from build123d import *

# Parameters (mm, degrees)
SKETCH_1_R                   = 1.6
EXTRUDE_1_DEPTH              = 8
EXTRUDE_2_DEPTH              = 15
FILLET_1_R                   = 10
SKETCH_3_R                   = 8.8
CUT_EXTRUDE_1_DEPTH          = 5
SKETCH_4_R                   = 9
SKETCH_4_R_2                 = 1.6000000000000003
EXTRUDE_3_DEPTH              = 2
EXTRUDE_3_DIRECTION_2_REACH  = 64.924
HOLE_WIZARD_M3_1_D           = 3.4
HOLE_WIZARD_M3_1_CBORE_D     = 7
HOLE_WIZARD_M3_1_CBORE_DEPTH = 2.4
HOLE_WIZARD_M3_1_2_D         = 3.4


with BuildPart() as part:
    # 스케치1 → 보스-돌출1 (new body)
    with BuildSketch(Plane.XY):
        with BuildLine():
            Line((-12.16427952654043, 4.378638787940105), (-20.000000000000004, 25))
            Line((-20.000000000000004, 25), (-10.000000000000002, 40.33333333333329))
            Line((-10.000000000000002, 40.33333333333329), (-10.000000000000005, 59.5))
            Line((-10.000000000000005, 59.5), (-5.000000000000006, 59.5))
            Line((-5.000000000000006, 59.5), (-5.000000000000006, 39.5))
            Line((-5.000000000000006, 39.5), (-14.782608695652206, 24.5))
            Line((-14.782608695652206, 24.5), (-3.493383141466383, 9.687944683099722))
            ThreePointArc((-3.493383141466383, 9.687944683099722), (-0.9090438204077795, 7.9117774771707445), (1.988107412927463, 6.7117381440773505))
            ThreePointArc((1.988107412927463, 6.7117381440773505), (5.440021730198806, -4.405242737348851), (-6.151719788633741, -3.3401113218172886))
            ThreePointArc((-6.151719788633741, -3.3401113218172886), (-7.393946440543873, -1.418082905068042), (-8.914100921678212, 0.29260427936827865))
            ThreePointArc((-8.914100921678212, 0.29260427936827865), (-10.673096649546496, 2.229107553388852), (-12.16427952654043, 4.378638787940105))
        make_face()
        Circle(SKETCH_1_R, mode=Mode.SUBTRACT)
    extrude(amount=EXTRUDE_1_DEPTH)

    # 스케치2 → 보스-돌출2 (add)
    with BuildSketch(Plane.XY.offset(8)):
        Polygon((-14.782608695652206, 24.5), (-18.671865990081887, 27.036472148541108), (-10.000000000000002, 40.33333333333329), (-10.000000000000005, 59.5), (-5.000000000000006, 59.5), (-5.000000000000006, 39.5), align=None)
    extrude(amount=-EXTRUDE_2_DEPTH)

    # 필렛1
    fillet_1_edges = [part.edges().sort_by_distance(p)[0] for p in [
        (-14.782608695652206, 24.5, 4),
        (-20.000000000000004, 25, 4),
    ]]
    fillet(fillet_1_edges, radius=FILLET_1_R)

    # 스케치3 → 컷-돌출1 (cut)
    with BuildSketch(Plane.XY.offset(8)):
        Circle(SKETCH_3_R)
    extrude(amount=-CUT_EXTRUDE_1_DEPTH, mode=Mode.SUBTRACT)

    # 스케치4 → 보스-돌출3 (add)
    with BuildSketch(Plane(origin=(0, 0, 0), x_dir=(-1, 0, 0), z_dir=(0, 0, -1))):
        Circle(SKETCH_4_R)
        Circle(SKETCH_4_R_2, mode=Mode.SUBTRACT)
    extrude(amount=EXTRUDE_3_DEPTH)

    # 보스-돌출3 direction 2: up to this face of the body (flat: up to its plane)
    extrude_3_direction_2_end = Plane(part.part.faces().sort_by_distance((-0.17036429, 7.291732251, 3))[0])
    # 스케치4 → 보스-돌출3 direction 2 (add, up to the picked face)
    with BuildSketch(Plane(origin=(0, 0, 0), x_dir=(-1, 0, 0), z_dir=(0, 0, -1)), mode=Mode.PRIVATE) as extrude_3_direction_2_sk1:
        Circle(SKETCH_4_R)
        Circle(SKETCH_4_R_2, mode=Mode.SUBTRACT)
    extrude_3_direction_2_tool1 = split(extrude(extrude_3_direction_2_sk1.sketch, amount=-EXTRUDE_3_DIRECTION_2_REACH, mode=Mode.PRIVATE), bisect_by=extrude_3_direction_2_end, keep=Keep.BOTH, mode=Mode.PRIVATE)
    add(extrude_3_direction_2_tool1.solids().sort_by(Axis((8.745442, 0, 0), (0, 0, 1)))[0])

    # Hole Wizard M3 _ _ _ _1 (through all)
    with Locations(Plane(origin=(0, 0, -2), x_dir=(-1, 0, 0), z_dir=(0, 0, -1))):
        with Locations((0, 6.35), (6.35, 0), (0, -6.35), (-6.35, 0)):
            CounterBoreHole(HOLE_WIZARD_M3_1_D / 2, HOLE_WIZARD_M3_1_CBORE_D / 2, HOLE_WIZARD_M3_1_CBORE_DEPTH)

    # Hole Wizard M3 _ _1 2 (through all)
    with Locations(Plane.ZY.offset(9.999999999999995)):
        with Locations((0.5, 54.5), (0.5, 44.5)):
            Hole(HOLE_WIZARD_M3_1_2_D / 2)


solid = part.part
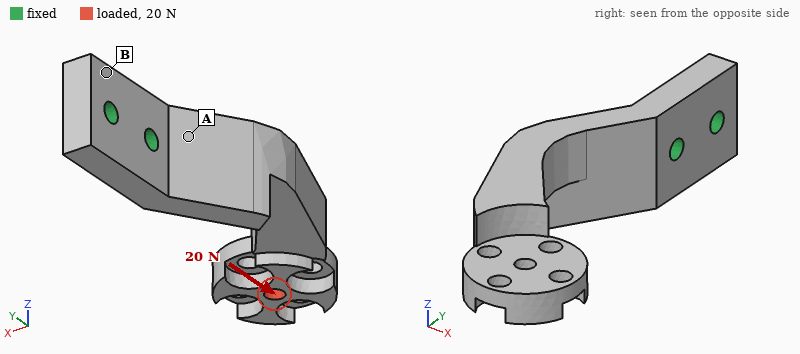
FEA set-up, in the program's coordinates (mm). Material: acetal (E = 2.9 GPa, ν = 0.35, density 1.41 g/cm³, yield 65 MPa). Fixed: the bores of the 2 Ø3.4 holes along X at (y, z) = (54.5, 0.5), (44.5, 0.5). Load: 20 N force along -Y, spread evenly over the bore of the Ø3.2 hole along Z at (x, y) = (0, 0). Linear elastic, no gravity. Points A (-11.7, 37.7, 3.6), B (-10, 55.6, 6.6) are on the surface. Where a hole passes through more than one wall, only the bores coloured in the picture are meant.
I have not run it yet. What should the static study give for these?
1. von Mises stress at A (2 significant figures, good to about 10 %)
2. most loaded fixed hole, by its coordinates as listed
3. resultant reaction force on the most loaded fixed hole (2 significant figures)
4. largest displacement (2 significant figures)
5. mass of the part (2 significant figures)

3.5 MPa
(44.5, 0.5)
16 N
0.87 mm
6.8 g
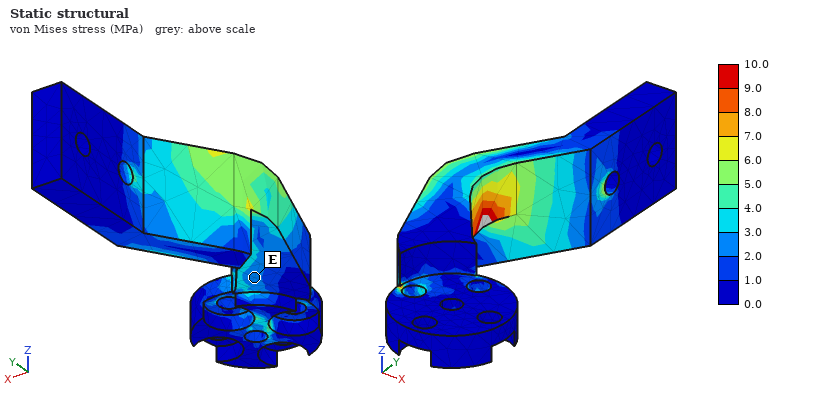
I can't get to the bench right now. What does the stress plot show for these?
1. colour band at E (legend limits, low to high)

2.0 to 3.0 MPa
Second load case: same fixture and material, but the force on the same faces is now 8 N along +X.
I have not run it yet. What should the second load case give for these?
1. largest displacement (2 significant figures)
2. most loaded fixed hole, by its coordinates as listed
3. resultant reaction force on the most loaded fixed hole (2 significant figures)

0.88 mm
(44.5, 0.5)
18 N
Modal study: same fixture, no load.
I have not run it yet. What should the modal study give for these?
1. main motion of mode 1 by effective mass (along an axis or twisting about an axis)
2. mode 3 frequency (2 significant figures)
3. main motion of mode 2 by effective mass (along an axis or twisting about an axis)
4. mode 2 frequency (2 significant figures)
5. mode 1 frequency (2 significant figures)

along X
1700 Hz
along Z
570 Hz
390 Hz
